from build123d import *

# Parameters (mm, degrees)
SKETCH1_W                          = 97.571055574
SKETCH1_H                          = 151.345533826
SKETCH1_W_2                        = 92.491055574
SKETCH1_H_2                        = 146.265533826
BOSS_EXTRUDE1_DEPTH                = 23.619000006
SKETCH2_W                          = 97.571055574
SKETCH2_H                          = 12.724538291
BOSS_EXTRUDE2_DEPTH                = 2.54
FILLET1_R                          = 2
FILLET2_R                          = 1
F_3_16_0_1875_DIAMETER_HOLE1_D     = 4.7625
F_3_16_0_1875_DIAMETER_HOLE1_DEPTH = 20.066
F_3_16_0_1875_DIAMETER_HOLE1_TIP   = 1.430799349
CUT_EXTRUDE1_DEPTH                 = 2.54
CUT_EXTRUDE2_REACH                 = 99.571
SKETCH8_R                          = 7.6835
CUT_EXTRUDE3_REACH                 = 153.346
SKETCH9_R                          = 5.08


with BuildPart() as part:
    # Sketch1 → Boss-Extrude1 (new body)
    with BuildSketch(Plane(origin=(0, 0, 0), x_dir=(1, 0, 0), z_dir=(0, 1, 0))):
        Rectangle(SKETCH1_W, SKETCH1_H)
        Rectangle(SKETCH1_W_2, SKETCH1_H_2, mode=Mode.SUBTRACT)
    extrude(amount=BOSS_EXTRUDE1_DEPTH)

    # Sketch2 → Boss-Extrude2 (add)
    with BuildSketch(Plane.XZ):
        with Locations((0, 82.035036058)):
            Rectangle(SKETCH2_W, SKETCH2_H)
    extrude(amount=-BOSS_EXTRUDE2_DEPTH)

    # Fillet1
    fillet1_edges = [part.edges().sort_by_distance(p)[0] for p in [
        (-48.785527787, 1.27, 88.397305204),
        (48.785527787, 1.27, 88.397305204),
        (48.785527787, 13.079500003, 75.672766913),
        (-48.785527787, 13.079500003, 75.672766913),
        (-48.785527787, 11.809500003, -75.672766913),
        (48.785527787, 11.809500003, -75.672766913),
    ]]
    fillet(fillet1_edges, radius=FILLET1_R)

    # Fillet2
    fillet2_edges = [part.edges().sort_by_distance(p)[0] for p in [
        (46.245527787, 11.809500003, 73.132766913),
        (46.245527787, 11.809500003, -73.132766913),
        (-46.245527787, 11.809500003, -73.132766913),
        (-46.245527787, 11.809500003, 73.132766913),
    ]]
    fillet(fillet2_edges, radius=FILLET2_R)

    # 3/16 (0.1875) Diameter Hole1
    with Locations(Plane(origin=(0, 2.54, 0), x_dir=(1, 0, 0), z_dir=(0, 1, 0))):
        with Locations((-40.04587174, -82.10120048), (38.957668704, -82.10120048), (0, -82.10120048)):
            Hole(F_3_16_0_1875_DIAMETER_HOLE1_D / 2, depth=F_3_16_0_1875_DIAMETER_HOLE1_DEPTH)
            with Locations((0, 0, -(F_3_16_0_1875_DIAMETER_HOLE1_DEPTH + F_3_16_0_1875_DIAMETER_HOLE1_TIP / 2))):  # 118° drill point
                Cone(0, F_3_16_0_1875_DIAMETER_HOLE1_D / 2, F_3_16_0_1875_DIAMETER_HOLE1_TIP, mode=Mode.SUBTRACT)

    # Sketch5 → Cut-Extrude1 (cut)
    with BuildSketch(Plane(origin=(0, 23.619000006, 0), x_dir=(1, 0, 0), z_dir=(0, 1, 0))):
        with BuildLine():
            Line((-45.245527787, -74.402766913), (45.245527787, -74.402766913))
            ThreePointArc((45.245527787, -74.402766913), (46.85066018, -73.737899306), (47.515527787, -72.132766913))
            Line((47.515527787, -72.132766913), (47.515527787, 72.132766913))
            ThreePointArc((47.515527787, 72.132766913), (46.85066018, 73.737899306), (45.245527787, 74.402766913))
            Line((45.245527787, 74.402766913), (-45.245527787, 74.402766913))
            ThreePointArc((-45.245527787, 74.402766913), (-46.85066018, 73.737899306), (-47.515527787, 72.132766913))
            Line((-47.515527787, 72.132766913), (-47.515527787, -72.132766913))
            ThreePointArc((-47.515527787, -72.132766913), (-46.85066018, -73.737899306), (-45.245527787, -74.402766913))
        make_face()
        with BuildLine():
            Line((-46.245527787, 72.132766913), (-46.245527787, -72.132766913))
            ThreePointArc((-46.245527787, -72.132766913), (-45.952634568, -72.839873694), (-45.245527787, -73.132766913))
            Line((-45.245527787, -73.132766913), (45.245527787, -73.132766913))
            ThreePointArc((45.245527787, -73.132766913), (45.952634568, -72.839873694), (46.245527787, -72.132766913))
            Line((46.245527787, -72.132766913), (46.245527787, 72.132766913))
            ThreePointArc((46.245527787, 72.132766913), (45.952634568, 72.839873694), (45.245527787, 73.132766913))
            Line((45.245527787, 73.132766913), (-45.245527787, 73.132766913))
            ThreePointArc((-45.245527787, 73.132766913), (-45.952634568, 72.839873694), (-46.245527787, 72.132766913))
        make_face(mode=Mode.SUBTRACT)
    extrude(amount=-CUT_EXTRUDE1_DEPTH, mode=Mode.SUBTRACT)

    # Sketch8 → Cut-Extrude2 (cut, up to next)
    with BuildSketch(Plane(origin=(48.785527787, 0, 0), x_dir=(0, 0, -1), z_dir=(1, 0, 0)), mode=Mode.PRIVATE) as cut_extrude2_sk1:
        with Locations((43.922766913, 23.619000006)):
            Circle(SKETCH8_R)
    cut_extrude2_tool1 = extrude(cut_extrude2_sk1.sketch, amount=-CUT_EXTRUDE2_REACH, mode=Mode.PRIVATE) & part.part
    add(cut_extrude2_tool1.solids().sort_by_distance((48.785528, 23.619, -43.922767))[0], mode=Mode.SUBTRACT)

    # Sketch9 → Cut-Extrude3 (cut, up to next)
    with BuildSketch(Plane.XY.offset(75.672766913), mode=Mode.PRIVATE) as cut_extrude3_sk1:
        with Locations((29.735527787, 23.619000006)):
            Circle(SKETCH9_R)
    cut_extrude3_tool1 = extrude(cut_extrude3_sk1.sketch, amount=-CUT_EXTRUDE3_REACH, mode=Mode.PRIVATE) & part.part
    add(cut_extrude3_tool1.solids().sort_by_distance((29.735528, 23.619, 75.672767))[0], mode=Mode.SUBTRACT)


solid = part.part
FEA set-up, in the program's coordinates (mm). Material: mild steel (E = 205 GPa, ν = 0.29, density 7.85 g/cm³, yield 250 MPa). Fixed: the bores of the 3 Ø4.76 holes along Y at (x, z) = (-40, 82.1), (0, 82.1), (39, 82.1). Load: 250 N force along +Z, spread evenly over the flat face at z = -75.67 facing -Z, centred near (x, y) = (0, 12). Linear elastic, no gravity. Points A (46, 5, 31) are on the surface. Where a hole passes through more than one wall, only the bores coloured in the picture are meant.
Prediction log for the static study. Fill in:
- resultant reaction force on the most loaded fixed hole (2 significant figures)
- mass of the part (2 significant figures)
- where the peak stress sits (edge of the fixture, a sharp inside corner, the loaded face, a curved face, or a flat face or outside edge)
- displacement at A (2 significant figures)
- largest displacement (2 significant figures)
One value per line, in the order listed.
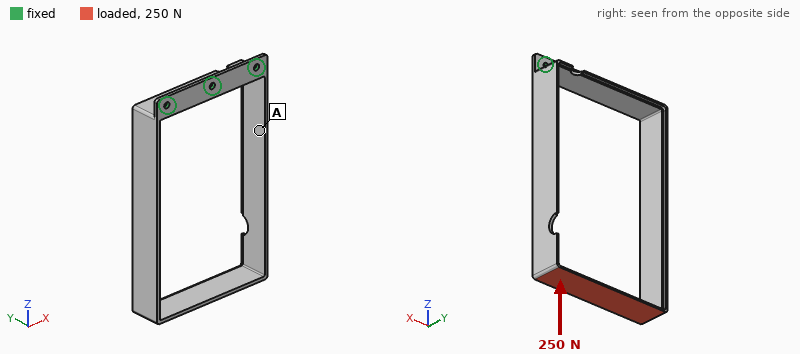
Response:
170 N
240 g
a flat face or outside edge
0.13 mm
0.45 mm
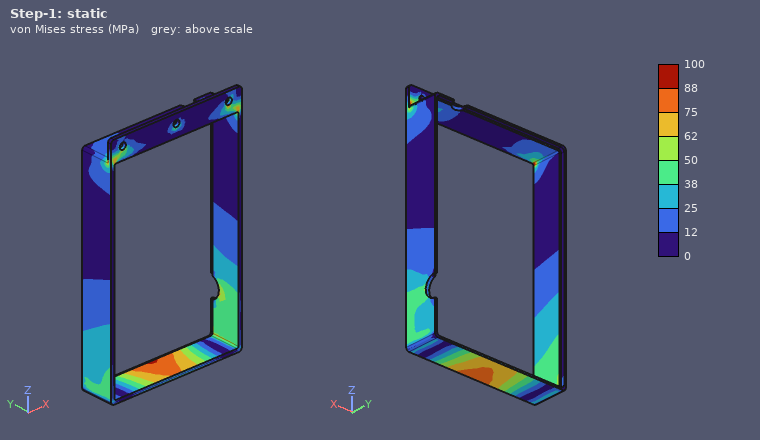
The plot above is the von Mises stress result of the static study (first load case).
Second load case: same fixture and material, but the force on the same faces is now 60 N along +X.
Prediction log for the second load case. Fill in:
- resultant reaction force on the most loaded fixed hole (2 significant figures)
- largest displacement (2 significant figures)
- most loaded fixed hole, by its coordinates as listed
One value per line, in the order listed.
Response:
130 N
1.8 mm
(0, 82.1)
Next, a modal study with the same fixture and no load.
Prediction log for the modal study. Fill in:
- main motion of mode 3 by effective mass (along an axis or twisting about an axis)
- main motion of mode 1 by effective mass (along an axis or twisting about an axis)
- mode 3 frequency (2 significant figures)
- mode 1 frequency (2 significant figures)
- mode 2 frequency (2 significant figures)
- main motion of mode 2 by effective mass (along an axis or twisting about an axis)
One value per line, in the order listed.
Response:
twisting about Z
along X
240 Hz
98 Hz
130 Hz
along Y
